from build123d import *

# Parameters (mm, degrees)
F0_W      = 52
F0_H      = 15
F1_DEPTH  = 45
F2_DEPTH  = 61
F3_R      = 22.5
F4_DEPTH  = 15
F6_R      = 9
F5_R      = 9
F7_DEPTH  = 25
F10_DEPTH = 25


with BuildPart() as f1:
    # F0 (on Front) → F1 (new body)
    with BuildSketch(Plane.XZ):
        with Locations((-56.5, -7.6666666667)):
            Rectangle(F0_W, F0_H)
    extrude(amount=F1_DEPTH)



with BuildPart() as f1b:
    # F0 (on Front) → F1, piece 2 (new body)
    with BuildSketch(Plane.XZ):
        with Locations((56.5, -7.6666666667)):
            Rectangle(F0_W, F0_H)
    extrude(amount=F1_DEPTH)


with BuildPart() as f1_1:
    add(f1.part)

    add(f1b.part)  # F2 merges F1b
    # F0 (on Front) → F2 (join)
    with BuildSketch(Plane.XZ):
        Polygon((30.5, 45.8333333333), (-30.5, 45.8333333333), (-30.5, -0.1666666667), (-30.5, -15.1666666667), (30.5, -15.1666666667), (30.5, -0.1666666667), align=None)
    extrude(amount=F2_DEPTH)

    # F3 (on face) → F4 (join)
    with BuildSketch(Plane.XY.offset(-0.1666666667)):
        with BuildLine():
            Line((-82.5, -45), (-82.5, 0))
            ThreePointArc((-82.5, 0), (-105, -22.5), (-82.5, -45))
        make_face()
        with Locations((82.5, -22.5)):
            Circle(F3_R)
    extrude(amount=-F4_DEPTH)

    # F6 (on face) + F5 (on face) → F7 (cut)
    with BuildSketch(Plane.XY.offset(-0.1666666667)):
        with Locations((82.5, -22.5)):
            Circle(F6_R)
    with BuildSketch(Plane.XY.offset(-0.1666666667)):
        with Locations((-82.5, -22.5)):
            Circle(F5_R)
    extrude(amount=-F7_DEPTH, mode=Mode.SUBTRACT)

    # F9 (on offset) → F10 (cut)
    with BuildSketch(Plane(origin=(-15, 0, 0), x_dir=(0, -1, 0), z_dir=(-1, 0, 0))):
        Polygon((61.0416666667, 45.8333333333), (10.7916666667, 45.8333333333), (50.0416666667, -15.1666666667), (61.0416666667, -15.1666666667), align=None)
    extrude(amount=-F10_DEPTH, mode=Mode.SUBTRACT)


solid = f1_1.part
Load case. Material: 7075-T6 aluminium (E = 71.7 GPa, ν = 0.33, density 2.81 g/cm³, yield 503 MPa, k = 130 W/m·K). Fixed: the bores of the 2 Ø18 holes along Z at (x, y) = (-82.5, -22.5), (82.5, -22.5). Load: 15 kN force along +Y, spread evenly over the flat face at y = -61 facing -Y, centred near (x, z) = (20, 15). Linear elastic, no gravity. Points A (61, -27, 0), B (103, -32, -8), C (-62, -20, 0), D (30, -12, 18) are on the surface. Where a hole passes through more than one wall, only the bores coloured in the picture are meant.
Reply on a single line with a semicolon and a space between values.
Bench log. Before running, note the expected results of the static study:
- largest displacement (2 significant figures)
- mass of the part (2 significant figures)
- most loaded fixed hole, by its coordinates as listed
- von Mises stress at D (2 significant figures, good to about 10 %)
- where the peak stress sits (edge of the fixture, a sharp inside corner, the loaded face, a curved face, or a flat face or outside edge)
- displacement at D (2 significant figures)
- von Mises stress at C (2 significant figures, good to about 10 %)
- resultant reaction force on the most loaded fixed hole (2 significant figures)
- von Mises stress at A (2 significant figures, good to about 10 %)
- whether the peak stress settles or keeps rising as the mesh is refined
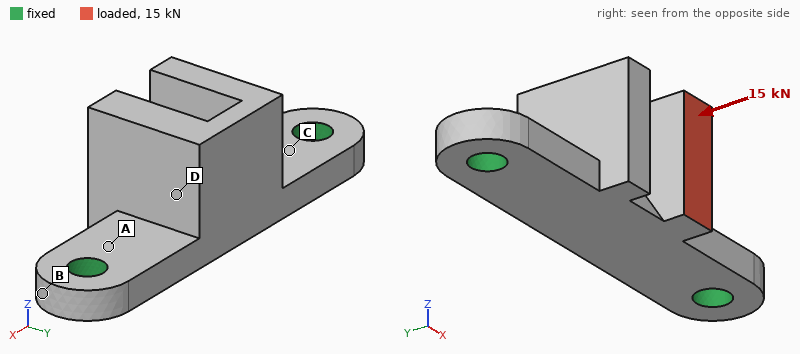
0.54 mm; 750 g; (82.5, -22.5); 26 MPa; edge of the fixture; 0.26 mm; 110 MPa; 9.8 kN; 130 MPa; keeps rising
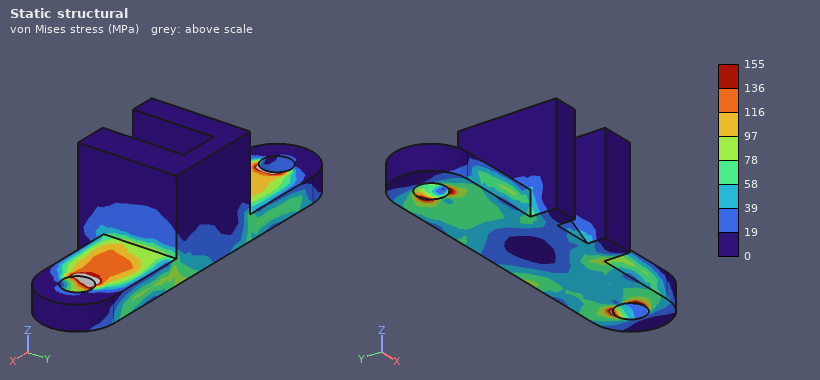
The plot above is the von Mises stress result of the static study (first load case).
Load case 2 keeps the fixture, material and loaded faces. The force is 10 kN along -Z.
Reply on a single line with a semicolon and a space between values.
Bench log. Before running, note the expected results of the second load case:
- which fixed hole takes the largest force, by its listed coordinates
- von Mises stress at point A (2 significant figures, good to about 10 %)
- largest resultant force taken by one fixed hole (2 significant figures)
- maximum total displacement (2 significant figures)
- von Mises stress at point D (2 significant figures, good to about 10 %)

(82.5, -22.5); 110 MPa; 7.2 kN; 0.61 mm; 23 MPa
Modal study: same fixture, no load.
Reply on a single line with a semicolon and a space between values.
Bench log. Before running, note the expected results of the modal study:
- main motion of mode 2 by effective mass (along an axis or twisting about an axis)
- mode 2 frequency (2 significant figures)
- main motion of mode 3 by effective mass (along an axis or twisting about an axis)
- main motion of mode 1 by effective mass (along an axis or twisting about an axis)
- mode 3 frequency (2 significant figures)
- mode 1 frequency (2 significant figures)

along Z; 2200 Hz; along X; along Y; 3500 Hz; 1400 Hz
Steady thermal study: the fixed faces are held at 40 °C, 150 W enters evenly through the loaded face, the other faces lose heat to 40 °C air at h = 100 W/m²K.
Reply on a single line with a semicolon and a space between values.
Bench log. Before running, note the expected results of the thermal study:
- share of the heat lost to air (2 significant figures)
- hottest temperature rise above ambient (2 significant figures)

50 %; 61 K
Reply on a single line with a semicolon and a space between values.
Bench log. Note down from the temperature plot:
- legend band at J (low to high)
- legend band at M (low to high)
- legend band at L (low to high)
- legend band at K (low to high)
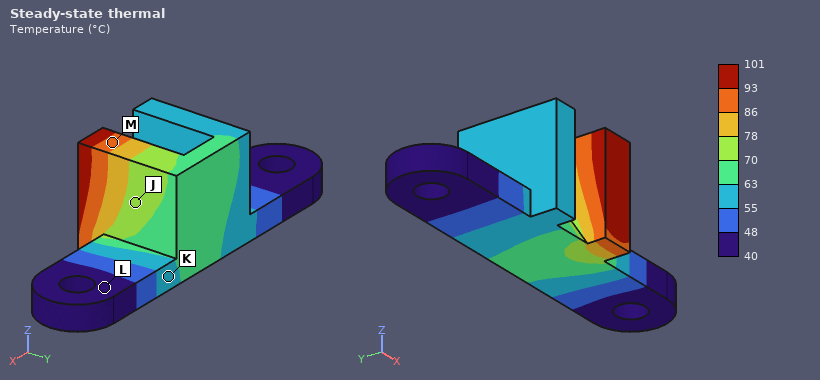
70 to 78 °C; 86 to 93 °C; 40 to 48 °C; 55 to 63 °C
